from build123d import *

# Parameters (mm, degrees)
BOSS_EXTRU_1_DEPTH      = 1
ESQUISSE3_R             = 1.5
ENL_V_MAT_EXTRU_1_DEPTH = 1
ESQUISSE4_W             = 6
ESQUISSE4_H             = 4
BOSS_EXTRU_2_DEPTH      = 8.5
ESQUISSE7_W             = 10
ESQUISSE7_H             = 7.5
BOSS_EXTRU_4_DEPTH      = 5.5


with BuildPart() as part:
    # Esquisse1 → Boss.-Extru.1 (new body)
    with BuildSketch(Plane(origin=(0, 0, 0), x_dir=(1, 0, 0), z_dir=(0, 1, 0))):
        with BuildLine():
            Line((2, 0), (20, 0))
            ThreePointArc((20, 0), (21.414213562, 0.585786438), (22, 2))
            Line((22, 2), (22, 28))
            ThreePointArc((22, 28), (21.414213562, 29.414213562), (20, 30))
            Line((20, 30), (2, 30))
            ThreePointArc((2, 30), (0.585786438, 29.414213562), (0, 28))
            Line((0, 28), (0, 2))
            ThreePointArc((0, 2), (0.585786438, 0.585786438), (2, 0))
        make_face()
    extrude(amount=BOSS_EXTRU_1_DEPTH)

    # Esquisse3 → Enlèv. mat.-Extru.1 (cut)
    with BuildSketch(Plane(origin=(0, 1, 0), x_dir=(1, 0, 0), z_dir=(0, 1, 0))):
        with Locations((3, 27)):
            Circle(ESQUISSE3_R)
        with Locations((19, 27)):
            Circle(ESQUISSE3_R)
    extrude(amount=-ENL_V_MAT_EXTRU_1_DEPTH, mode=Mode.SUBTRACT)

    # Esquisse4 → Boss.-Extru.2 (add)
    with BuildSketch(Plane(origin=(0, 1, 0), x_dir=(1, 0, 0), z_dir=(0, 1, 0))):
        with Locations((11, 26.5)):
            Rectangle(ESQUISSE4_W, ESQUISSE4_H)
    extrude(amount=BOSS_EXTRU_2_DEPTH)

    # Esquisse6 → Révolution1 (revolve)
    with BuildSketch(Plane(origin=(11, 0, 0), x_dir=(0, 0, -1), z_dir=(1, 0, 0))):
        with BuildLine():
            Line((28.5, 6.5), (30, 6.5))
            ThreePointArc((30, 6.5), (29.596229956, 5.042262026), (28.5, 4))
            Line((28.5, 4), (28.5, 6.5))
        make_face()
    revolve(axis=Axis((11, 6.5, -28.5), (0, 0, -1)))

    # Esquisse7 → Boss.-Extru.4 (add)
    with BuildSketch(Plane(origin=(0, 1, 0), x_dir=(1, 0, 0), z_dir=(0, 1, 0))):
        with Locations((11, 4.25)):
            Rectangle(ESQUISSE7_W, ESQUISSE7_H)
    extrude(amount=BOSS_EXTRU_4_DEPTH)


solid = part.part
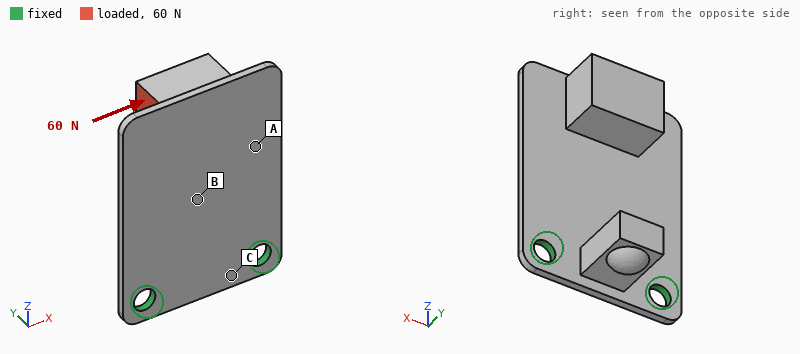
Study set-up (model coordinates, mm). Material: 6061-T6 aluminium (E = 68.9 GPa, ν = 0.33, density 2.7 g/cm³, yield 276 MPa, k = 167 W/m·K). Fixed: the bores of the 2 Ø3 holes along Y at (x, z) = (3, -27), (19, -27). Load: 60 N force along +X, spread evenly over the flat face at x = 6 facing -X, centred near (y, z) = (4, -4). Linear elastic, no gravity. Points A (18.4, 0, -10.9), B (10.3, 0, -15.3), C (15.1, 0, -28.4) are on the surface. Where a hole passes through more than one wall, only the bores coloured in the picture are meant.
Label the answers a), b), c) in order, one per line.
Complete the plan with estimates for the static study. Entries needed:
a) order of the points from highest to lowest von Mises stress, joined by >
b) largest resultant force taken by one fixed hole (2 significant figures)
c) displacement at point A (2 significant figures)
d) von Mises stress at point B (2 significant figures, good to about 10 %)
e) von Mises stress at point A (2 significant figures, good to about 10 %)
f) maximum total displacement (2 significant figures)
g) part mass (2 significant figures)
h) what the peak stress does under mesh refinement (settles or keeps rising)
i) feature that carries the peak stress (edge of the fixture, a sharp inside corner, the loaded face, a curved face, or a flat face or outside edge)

a) B > A > C
b) 85 N
c) 0.064 mm
d) 31 MPa
e) 20 MPa
f) 0.12 mm
g) 3.4 g
h) keeps rising
i) edge of the fixture
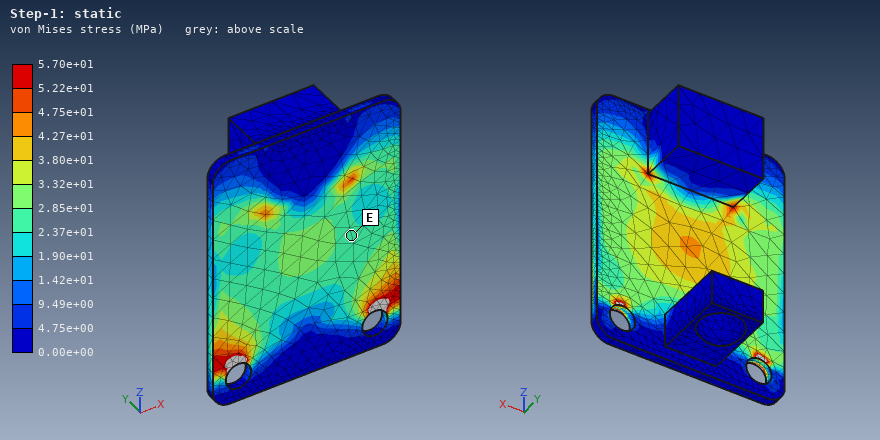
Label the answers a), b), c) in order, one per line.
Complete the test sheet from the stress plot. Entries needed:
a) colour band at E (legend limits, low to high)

a) 2.37e+01 to 2.85e+01 MPa
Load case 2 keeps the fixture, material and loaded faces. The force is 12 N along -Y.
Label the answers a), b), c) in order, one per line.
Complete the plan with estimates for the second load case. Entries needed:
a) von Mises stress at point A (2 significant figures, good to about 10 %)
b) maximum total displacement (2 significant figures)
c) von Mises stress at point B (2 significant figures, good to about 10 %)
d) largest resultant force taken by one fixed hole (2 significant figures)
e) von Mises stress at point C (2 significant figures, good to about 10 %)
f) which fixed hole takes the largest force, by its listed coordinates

a) 26 MPa
b) 0.45 mm
c) 35 MPa
d) 9.9 N
e) 27 MPa
f) (3, -27)
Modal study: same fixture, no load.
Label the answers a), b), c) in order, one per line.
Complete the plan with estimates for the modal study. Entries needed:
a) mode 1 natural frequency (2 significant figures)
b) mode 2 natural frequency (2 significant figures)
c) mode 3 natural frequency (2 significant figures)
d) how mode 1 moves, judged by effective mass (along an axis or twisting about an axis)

a) 710 Hz
b) 2900 Hz
c) 5100 Hz
d) along Y
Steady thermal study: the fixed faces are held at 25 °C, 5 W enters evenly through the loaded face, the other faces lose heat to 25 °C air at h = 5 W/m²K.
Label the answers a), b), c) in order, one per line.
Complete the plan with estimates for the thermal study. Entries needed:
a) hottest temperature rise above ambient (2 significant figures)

a) 33 K
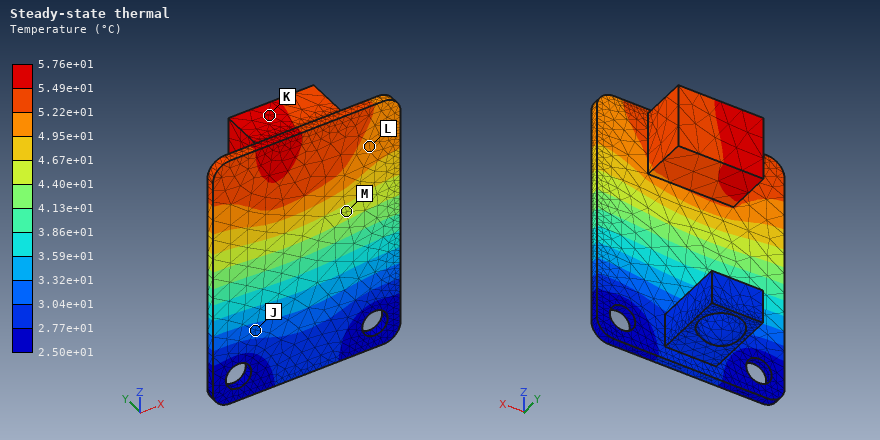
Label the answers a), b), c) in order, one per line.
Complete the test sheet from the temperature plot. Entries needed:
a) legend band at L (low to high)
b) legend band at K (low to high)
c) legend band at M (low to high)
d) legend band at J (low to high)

a) 4.95e+01 to 5.22e+01 °C
b) 5.49e+01 to 5.76e+01 °C
c) 4.40e+01 to 4.67e+01 °C
d) 3.04e+01 to 3.32e+01 °C
